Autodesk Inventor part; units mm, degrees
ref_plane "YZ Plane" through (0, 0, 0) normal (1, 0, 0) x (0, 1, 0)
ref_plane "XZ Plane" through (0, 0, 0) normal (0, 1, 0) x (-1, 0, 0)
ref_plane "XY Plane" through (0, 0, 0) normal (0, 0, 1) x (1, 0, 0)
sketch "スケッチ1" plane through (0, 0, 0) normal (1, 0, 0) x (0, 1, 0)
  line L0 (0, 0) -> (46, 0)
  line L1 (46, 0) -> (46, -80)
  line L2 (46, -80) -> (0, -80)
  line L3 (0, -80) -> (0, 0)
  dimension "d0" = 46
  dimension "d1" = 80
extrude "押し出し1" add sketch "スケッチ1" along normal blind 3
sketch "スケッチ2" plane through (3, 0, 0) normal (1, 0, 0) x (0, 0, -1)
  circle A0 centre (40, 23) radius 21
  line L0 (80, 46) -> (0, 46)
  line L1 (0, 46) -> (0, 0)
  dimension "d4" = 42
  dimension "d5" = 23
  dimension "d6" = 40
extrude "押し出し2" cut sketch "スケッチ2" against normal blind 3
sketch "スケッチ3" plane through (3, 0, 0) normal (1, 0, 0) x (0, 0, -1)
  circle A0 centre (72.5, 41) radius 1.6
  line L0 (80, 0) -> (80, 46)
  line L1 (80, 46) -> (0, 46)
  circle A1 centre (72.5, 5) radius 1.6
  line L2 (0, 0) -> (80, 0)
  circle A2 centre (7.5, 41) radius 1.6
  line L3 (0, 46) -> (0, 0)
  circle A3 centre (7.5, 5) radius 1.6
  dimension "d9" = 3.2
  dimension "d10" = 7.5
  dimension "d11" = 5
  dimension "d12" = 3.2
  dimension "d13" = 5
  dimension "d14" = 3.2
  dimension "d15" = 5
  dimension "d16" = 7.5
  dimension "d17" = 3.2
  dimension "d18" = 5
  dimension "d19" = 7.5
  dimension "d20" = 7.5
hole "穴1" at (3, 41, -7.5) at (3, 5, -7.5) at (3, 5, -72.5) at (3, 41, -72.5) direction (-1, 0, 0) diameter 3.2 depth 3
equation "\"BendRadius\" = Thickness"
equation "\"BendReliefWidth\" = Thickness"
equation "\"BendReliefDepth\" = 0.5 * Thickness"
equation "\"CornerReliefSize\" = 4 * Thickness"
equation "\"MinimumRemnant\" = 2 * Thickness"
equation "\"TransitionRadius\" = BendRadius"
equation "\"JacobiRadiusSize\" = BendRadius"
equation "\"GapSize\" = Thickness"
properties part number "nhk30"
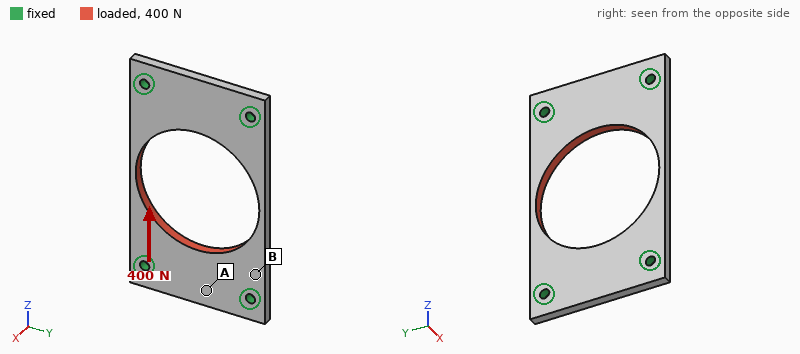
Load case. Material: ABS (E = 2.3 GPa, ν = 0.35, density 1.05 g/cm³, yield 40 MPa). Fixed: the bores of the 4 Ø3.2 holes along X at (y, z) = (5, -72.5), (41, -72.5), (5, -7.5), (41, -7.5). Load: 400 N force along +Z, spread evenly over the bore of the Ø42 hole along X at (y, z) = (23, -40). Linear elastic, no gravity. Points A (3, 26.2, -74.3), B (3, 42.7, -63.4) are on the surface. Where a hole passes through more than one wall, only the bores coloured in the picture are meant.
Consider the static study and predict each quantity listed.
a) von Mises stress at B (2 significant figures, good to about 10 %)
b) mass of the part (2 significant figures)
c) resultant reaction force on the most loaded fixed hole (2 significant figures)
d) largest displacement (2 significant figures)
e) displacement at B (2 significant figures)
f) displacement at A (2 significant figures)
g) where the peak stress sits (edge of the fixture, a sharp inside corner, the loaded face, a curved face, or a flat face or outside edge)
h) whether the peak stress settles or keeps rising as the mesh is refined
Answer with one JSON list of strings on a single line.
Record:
["2.4 MPa", "7.1 g", "100 N", "33 µm", "10 µm", "20 µm", "edge of the fixture", "keeps rising"]
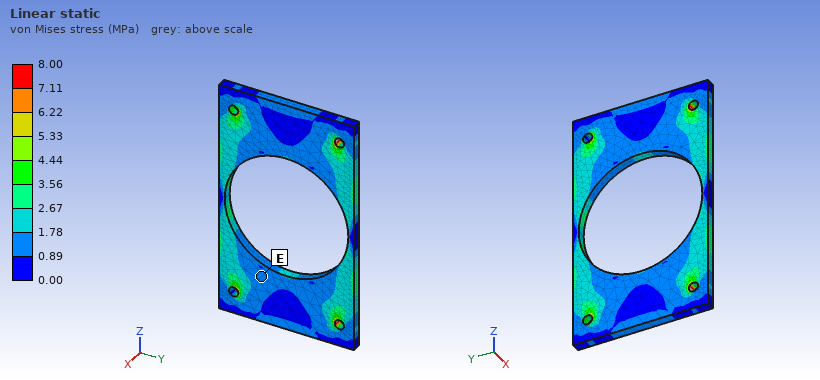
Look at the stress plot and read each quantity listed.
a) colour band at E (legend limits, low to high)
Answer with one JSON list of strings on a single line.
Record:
["0.89 to 1.78 MPa"]
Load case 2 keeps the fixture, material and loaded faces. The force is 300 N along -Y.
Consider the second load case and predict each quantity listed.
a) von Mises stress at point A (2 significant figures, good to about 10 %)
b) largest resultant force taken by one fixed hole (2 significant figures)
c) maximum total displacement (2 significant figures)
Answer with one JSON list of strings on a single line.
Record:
["1.6 MPa", "79 N", "0.21 mm"]
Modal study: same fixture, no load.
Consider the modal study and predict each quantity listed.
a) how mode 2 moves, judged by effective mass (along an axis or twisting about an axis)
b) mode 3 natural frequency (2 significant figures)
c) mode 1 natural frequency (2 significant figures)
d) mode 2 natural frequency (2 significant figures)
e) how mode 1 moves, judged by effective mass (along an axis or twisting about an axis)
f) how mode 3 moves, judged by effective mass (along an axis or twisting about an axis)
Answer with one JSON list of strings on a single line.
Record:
["twisting about Z", "2500 Hz", "1500 Hz", "1700 Hz", "along X", "twisting about Y"]
